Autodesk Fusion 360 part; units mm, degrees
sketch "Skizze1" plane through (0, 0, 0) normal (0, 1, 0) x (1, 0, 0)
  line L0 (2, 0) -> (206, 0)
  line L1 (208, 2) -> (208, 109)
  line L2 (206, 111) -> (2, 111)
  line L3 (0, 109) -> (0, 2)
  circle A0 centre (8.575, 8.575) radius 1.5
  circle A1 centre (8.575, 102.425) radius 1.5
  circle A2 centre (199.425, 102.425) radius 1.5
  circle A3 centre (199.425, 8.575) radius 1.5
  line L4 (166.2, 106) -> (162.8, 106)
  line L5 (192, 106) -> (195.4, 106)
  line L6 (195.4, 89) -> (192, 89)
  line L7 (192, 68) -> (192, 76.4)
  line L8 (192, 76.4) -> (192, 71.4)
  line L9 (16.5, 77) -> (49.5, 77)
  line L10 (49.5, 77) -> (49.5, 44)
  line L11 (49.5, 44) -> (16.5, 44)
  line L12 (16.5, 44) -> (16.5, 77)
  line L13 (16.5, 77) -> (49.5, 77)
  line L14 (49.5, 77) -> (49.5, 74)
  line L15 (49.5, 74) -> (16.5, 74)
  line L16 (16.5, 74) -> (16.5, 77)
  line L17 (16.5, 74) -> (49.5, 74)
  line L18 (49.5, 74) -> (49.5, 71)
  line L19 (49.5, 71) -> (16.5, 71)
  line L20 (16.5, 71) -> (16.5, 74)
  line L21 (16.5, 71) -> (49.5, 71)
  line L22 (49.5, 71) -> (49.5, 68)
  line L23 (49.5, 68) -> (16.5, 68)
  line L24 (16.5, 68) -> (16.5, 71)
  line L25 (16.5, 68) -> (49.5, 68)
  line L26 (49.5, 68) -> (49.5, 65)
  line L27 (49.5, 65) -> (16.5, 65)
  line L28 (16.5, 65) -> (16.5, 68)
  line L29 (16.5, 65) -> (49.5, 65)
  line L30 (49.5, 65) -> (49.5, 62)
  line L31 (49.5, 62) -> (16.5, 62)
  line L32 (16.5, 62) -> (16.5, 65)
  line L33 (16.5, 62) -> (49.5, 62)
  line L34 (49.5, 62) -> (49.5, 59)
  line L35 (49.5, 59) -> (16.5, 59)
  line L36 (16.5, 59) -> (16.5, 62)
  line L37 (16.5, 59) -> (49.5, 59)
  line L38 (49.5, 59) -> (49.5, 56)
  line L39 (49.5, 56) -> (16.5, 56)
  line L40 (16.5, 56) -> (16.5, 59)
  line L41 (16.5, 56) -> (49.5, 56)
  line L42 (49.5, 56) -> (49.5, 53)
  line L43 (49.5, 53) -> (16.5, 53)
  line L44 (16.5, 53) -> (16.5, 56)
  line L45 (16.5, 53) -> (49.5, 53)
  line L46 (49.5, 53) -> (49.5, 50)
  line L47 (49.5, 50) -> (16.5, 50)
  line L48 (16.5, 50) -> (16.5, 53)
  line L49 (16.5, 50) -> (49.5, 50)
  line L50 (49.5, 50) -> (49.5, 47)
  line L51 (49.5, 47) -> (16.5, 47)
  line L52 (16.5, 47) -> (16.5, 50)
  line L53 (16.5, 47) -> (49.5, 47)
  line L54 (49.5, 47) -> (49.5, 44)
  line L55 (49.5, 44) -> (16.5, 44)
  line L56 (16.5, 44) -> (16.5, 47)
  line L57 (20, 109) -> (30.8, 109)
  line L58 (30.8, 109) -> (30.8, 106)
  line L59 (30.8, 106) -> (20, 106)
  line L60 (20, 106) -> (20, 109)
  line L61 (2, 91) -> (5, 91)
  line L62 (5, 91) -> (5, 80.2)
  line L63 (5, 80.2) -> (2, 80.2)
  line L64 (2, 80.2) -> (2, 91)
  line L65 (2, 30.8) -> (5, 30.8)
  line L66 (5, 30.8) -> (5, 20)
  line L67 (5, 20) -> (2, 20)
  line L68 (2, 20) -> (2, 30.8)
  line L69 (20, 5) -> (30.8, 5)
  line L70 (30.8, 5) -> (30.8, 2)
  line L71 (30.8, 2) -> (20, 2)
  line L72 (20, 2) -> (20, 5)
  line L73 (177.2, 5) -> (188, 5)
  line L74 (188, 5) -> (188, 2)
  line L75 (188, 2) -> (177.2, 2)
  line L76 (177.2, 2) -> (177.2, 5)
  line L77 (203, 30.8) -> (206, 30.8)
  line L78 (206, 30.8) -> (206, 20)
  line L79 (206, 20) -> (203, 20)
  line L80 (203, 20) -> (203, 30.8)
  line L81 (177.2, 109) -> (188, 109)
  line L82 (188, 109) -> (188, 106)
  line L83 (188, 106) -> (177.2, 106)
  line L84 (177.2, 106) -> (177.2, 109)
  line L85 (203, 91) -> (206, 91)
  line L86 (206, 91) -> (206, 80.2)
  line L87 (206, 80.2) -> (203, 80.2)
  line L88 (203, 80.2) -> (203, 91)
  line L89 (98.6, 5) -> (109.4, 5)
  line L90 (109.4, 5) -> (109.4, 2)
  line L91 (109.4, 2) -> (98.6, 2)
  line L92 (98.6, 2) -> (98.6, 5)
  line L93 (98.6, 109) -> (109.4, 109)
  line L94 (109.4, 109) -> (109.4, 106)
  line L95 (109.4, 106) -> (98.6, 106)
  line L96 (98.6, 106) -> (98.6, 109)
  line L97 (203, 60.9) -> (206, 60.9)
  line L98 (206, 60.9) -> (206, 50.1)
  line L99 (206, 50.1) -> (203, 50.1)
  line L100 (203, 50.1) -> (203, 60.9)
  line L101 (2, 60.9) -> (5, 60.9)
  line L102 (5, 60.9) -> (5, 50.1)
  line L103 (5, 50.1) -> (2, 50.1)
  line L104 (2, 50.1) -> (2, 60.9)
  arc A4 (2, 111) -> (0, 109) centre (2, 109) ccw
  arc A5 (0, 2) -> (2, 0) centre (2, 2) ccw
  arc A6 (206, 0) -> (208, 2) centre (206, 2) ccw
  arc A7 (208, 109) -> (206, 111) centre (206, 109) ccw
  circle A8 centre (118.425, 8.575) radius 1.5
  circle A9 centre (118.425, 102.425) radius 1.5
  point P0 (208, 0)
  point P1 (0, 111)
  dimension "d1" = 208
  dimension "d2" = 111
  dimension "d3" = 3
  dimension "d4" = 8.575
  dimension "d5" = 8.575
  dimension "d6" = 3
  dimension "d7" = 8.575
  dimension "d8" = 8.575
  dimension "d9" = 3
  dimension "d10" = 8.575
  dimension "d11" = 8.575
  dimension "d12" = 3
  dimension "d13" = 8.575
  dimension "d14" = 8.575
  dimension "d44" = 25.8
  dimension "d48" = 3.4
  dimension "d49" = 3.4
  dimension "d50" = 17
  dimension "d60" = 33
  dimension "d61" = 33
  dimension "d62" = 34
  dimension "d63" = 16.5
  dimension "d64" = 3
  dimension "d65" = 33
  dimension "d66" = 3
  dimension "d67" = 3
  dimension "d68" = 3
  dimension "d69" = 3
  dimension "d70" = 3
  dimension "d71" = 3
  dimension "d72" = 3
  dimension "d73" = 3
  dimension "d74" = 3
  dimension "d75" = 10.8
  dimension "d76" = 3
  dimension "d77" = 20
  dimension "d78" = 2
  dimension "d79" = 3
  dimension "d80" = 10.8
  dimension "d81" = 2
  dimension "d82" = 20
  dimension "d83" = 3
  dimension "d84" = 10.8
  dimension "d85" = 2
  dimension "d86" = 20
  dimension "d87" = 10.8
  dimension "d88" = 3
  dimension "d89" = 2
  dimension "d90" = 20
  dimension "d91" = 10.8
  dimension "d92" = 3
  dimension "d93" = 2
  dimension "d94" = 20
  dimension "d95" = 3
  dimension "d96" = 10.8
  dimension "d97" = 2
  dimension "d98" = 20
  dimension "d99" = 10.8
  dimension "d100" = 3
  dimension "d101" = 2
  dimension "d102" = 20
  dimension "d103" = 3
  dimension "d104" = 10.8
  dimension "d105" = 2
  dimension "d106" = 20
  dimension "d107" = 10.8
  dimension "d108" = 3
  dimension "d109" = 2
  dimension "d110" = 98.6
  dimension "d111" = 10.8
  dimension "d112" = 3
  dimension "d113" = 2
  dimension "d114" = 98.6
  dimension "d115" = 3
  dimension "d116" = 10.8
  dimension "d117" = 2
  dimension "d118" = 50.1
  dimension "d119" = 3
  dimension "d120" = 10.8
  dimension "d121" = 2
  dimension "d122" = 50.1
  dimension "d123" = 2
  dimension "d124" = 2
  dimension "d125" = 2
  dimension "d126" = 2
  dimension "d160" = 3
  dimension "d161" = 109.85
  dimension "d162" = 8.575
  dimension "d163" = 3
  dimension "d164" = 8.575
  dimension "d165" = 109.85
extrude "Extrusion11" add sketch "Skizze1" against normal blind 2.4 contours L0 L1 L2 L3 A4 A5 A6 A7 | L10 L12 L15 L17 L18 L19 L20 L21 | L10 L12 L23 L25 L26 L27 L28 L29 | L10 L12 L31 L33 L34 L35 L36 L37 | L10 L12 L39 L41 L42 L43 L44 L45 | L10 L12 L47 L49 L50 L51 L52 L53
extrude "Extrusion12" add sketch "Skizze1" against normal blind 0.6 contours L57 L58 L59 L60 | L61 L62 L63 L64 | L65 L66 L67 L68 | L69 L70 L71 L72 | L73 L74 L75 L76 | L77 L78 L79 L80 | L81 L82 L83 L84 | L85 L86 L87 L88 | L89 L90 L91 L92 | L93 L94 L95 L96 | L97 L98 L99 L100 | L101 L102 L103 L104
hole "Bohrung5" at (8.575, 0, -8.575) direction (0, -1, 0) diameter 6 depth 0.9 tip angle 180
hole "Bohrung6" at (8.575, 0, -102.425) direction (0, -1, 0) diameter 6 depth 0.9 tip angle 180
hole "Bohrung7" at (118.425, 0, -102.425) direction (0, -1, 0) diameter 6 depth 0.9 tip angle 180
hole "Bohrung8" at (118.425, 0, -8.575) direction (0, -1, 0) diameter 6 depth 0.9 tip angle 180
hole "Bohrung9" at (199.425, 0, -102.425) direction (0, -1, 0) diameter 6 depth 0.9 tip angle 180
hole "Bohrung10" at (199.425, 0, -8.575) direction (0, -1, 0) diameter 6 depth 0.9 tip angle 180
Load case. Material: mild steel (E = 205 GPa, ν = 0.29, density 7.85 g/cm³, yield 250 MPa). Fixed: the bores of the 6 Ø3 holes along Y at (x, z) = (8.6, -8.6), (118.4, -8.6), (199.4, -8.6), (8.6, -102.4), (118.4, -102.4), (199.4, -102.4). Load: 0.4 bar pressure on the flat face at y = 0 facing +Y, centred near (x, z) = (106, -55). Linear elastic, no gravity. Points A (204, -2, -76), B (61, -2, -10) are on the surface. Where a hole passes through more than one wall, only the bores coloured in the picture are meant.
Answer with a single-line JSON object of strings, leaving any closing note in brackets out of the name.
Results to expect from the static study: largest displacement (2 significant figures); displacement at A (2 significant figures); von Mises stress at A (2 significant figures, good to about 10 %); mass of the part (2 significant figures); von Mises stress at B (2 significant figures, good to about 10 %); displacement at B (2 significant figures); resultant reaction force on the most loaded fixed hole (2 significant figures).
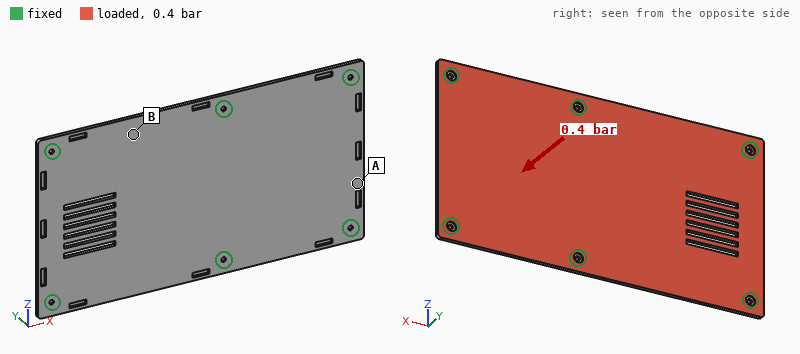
{"largest displacement": "0.17 mm", "displacement at A": "0.042 mm", "von Mises stress at A": "11 MPa", "mass of the part": "420 g", "von Mises stress at B": "28 MPa", "displacement at B": "0.11 mm", "resultant reaction force on the most loaded fixed hole": "380 N"}
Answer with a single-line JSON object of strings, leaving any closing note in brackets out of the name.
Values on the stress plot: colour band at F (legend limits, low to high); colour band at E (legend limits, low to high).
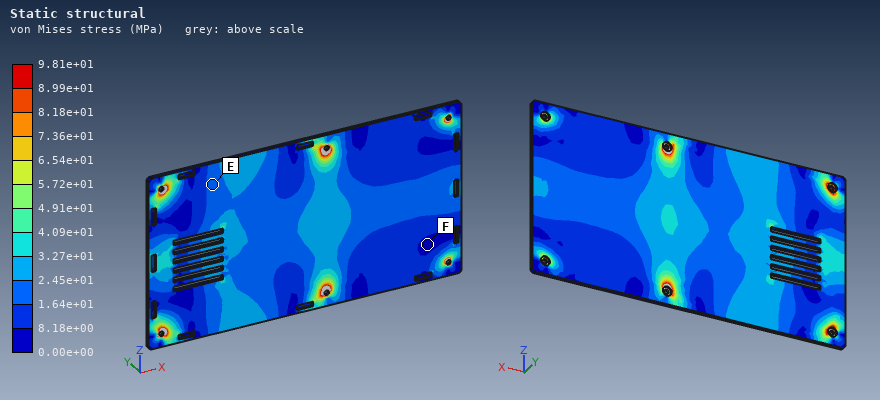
{"colour band at F": "0.00e+00 to 8.18e+00 MPa", "colour band at E": "1.64e+01 to 2.45e+01 MPa"}
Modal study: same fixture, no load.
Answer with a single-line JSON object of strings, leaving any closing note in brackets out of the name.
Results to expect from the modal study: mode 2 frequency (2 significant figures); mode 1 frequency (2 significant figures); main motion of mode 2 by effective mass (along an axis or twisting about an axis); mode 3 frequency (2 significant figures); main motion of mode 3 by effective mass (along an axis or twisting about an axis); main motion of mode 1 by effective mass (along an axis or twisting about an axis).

{"mode 2 frequency": "940 Hz", "mode 1 frequency": "680 Hz", "main motion of mode 2 by effective mass": "along Y", "mode 3 frequency": "1100 Hz", "main motion of mode 3 by effective mass": "twisting about X", "main motion of mode 1 by effective mass": "along Y"}
